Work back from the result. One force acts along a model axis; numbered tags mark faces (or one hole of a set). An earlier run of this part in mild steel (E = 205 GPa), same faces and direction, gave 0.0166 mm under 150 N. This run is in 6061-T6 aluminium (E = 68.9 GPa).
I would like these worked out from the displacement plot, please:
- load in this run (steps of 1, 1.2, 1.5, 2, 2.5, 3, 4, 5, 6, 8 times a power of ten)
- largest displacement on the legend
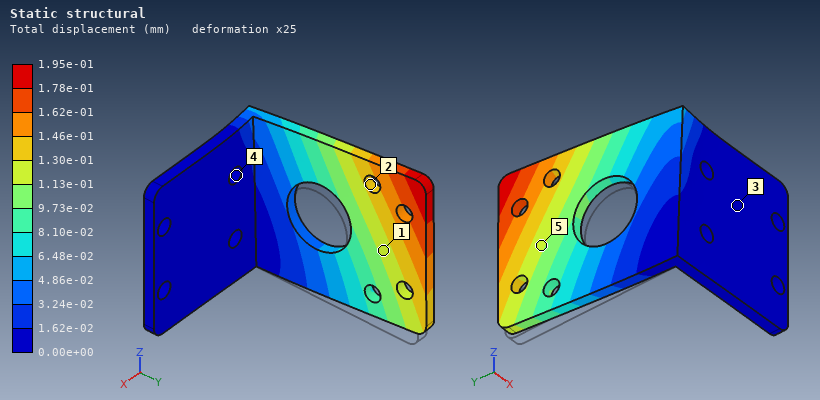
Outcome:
600 N
1.95e-01 mm
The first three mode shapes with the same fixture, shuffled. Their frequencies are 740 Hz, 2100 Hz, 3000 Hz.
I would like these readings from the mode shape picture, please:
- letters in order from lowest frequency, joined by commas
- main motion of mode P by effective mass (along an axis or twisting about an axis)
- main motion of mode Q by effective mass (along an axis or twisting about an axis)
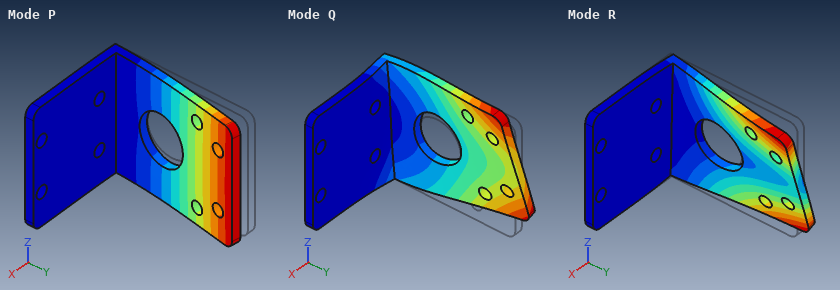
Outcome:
P, R, Q
along X
along Z
